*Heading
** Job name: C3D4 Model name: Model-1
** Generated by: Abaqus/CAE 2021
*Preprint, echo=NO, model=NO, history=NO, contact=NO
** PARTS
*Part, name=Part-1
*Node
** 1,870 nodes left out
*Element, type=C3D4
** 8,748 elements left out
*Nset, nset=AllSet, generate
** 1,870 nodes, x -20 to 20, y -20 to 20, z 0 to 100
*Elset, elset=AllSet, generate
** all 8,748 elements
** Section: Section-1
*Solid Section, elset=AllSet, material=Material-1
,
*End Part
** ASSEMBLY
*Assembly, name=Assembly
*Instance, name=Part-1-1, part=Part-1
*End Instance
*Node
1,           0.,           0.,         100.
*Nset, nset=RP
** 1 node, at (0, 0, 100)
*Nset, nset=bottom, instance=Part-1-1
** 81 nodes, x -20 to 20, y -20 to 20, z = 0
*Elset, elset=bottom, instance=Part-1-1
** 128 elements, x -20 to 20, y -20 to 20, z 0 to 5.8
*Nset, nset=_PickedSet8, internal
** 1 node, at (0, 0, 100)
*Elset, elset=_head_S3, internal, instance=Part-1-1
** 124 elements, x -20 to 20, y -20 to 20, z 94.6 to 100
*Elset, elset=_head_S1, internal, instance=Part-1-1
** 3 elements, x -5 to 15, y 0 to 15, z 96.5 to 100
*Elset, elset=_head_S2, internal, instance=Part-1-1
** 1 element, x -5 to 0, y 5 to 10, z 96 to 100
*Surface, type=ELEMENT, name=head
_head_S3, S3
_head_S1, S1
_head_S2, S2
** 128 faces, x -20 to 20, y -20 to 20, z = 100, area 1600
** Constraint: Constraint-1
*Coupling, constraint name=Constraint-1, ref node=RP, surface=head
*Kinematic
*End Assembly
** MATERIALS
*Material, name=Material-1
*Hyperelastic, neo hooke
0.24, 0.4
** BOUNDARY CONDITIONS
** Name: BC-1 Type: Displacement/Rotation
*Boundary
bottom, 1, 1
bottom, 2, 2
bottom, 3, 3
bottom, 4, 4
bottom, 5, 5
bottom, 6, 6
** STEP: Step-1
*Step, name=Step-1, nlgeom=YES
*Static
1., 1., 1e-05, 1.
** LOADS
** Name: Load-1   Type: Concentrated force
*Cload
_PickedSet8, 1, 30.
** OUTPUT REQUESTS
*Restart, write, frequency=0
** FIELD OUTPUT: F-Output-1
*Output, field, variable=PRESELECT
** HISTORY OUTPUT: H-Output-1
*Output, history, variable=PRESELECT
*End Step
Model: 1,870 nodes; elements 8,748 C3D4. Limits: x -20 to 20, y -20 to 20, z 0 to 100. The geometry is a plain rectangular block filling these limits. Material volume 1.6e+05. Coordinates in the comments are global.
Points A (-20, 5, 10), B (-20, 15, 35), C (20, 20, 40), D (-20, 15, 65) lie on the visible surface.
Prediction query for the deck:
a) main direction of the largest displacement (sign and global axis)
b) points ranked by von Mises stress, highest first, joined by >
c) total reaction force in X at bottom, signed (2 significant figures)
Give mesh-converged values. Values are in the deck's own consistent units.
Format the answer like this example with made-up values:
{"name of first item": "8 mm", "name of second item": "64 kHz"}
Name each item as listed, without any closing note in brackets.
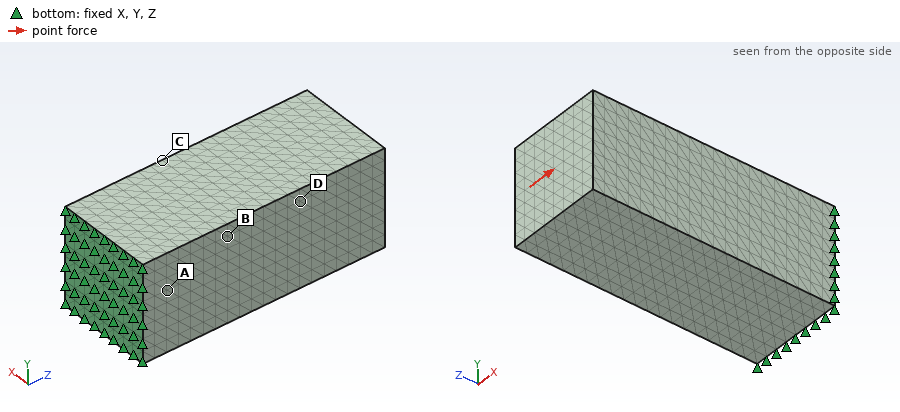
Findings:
{"main direction of the largest displacement": "+X", "points ranked by von Mises stress, highest first, joined by >": "A > B > C > D", "total reaction force in X at bottom, signed": "-30"}
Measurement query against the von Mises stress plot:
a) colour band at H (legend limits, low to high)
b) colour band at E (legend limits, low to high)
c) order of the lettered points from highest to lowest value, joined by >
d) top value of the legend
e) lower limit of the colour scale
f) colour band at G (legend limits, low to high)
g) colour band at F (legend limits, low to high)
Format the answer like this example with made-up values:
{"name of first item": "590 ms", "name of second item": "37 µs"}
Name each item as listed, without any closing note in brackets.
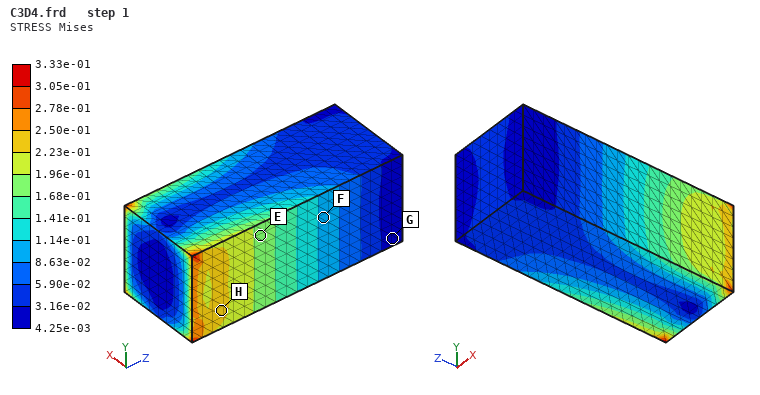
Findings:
{"colour band at H": "2.23e-01 to 2.50e-01", "colour band at E": "1.68e-01 to 1.96e-01", "order of the lettered points from highest to lowest value, joined by >": "H > E > F > G", "top value of the legend": "3.33e-01", "lower limit of the colour scale": "4.25e-03", "colour band at G": "4.25e-03 to 3.16e-02", "colour band at F": "8.63e-02 to 1.14e-01"}
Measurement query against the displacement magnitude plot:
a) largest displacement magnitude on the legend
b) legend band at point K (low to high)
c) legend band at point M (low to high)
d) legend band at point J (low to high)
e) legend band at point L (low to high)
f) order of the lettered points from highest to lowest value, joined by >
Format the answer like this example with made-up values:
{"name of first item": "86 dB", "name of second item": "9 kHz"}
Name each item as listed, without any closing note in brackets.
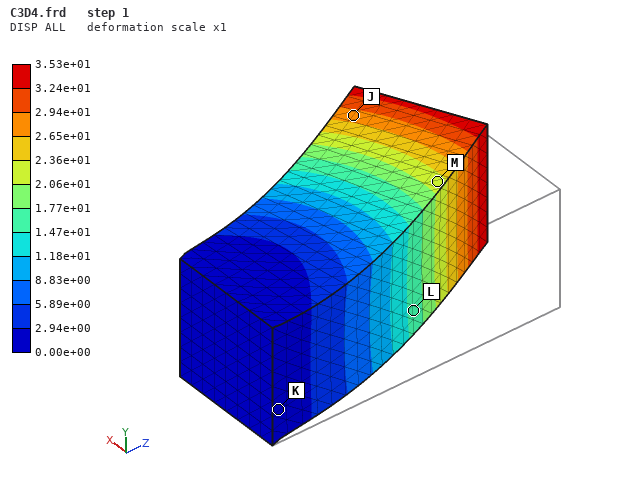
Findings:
{"largest displacement magnitude on the legend": "3.53e+01", "legend band at point K": "0.00e+00 to 2.94e+00", "legend band at point M": "2.06e+01 to 2.36e+01", "legend band at point J": "2.65e+01 to 2.94e+01", "legend band at point L": "1.47e+01 to 1.77e+01", "order of the lettered points from highest to lowest value, joined by >": "J > M > L > K"}
